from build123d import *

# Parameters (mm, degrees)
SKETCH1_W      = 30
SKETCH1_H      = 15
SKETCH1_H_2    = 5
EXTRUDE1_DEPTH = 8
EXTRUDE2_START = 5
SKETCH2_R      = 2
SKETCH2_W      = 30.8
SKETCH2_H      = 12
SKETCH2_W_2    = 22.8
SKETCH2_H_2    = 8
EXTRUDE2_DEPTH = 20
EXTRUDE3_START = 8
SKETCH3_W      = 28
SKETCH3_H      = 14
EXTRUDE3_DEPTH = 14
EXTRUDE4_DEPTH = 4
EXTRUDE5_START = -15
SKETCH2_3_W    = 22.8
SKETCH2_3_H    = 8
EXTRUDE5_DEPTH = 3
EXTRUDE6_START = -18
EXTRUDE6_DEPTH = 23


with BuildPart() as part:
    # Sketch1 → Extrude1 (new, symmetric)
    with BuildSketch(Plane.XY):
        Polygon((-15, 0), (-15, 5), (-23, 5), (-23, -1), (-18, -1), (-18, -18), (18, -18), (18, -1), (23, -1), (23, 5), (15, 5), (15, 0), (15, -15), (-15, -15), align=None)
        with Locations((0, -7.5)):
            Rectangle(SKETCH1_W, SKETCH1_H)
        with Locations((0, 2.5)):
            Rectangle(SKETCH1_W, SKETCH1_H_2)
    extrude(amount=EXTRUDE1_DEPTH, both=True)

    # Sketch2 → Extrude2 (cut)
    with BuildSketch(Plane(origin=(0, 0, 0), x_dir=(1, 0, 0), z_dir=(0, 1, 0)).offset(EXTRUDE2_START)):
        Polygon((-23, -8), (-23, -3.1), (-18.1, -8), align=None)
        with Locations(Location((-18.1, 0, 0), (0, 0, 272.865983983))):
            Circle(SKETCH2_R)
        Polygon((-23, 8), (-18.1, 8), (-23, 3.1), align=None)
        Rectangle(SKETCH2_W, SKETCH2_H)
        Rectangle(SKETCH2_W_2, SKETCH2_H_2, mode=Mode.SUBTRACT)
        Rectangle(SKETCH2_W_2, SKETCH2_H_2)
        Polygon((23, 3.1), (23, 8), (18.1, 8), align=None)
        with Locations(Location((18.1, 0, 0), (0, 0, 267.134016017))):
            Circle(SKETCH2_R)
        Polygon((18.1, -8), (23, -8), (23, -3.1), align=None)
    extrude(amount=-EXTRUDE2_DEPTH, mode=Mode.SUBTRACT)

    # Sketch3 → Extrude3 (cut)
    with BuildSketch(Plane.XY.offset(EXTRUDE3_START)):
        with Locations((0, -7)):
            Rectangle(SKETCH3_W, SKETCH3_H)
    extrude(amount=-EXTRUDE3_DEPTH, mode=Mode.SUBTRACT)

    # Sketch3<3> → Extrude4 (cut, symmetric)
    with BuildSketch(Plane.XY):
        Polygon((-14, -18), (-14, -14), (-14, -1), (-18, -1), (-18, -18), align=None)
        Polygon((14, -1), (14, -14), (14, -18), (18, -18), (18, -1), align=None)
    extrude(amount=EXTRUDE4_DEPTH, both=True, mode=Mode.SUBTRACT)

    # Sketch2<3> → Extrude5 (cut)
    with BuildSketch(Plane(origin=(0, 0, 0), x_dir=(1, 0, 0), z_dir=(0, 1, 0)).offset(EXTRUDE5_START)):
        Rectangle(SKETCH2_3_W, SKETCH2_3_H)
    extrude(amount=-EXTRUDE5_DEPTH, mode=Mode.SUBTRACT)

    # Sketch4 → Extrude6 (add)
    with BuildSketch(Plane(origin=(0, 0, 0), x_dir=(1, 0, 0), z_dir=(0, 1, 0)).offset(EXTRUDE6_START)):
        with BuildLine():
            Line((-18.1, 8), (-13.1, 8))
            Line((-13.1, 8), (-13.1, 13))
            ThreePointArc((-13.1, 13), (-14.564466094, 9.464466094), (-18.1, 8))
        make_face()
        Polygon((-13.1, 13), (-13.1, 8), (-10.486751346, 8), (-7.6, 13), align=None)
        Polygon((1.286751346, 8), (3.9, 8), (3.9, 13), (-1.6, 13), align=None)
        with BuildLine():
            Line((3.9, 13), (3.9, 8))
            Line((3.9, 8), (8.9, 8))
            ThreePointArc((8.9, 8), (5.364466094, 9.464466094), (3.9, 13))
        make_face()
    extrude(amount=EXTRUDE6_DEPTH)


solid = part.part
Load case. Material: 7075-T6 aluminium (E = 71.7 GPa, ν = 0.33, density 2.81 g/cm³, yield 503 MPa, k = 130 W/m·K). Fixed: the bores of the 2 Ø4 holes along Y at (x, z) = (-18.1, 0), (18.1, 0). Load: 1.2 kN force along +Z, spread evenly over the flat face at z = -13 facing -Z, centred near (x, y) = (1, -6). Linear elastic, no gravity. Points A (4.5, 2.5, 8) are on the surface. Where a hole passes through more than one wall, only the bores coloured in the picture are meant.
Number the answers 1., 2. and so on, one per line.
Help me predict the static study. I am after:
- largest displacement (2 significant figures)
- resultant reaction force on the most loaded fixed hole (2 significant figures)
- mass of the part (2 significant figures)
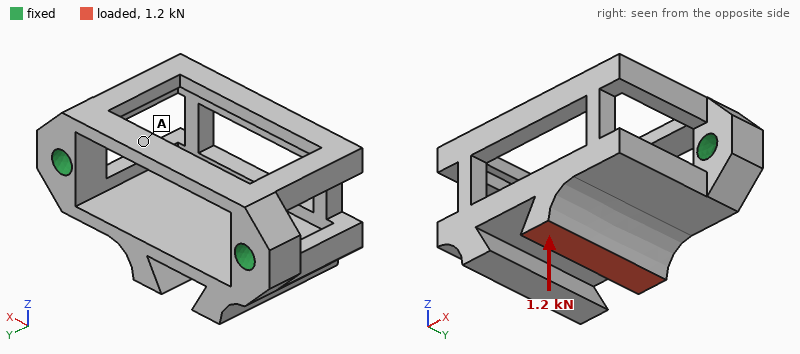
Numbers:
1. 0.21 mm
2. 750 N
3. 15 g
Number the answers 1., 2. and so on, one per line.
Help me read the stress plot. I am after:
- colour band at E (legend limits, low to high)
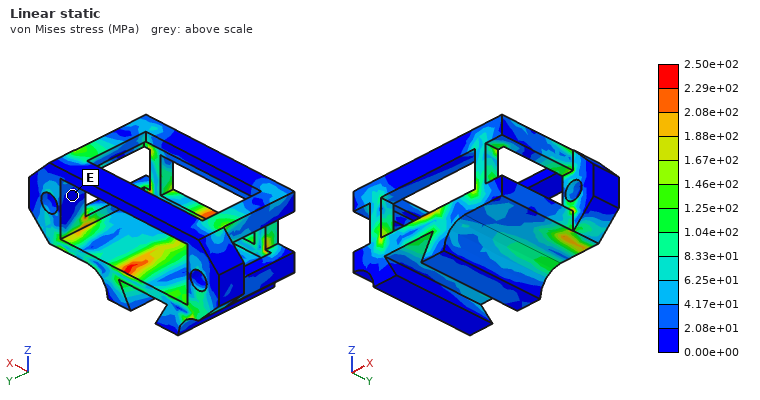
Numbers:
1. 0.00e+00 to 2.08e+01 MPa
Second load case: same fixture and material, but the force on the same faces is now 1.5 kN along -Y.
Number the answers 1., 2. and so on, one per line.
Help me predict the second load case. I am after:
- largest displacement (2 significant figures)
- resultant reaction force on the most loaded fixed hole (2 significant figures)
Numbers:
1. 0.21 mm
2. 900 N
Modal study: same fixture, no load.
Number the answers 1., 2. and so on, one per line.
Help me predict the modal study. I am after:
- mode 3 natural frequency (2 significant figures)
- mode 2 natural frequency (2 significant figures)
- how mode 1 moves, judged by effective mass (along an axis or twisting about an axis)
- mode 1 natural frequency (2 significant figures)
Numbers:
1. 8500 Hz
2. 7900 Hz
3. along Z
4. 4700 Hz
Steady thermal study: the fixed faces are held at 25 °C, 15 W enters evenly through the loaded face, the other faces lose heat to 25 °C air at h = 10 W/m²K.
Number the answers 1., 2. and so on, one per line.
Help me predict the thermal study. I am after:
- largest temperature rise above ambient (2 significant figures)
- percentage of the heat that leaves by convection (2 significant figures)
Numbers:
1. 37 K
2. 4.5 %
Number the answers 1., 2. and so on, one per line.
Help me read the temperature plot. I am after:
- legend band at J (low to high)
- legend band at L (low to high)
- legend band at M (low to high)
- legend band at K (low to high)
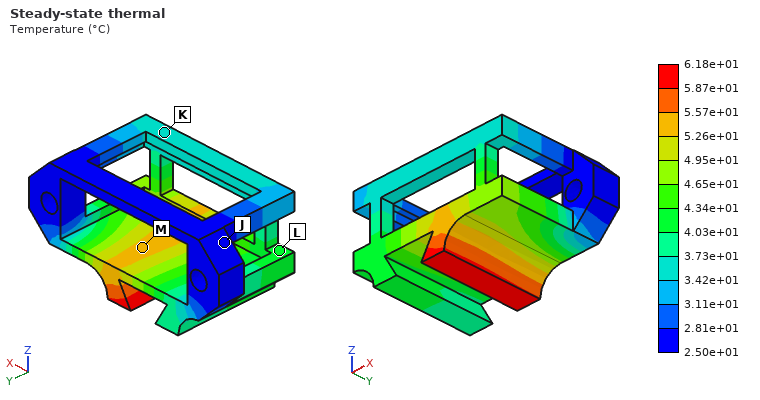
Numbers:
1. 2.50e+01 to 2.81e+01 °C
2. 4.03e+01 to 4.34e+01 °C
3. 5.26e+01 to 5.57e+01 °C
4. 3.42e+01 to 3.73e+01 °C
